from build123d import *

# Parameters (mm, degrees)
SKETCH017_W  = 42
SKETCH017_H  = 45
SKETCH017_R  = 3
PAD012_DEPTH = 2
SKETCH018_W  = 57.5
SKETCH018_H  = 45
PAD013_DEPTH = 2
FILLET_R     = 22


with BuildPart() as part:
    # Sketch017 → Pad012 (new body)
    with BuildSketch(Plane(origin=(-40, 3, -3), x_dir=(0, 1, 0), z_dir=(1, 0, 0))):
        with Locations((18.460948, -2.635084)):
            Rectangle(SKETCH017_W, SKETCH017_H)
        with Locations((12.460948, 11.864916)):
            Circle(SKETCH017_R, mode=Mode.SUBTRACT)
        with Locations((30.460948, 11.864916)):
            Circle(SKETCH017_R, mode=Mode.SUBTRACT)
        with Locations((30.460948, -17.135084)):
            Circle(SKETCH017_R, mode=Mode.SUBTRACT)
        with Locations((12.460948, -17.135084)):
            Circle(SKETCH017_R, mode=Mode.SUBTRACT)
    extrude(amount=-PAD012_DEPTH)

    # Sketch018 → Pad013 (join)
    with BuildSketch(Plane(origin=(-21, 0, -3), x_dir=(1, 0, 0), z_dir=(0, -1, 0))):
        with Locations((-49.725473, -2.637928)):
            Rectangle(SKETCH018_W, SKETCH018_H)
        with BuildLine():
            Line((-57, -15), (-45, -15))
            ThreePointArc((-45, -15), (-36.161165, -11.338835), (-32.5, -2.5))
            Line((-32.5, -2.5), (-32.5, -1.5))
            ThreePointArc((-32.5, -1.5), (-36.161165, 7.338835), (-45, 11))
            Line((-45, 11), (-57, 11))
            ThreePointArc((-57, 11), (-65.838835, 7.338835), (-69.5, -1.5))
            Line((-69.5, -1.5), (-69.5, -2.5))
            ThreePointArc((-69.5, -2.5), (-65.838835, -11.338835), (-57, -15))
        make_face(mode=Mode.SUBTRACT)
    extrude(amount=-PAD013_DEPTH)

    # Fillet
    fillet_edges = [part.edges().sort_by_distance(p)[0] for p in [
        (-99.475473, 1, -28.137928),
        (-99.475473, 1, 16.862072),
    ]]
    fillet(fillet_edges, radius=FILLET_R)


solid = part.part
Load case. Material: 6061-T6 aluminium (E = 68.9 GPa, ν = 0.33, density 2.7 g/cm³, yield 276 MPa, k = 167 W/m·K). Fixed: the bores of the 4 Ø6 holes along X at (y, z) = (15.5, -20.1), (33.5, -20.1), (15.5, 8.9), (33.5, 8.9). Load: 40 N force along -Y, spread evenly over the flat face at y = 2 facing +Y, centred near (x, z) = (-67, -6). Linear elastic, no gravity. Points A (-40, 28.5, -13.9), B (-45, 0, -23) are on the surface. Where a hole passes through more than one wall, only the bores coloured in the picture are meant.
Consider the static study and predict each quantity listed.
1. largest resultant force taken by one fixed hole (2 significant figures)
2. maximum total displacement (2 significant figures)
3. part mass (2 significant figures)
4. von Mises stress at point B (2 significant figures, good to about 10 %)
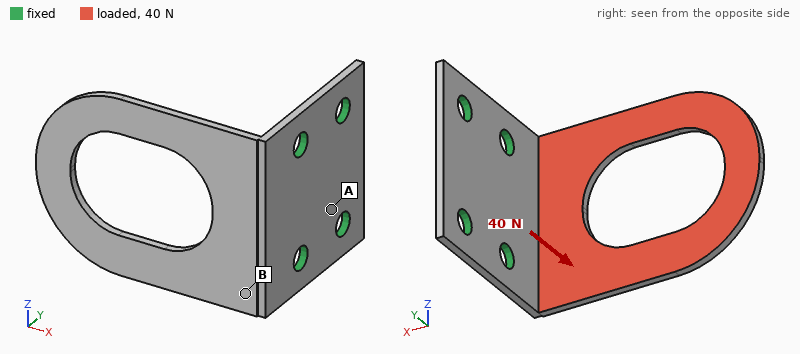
17 N
0.96 mm
18 g
27 MPa
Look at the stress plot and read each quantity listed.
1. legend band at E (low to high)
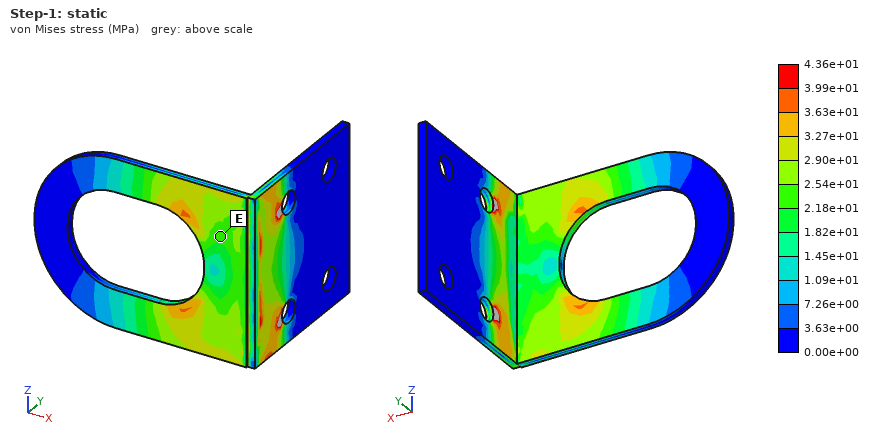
2.18e+01 to 2.54e+01 MPa
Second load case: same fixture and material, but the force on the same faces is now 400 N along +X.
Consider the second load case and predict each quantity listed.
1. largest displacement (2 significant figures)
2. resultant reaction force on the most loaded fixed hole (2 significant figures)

0.48 mm
220 N
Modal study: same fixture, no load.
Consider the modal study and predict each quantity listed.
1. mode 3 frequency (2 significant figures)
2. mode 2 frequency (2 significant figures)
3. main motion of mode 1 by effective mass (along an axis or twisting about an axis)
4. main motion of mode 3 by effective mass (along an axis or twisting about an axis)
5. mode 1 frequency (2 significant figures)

1800 Hz
1200 Hz
along Y
along Z
440 Hz
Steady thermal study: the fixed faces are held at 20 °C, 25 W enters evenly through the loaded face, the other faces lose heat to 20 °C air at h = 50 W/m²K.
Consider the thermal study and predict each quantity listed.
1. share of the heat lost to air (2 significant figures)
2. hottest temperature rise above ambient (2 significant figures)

24 %
75 K
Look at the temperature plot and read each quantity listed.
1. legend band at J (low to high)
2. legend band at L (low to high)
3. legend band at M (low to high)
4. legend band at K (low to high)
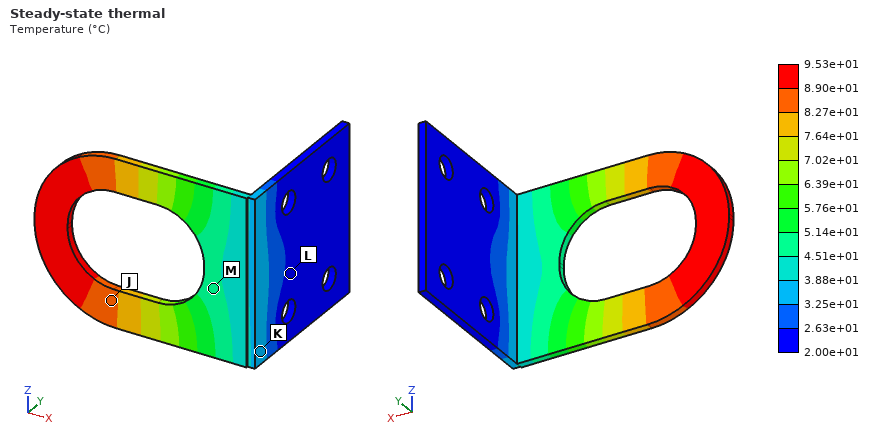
8.27e+01 to 8.90e+01 °C
2.00e+01 to 2.63e+01 °C
4.51e+01 to 5.14e+01 °C
3.25e+01 to 3.88e+01 °C
